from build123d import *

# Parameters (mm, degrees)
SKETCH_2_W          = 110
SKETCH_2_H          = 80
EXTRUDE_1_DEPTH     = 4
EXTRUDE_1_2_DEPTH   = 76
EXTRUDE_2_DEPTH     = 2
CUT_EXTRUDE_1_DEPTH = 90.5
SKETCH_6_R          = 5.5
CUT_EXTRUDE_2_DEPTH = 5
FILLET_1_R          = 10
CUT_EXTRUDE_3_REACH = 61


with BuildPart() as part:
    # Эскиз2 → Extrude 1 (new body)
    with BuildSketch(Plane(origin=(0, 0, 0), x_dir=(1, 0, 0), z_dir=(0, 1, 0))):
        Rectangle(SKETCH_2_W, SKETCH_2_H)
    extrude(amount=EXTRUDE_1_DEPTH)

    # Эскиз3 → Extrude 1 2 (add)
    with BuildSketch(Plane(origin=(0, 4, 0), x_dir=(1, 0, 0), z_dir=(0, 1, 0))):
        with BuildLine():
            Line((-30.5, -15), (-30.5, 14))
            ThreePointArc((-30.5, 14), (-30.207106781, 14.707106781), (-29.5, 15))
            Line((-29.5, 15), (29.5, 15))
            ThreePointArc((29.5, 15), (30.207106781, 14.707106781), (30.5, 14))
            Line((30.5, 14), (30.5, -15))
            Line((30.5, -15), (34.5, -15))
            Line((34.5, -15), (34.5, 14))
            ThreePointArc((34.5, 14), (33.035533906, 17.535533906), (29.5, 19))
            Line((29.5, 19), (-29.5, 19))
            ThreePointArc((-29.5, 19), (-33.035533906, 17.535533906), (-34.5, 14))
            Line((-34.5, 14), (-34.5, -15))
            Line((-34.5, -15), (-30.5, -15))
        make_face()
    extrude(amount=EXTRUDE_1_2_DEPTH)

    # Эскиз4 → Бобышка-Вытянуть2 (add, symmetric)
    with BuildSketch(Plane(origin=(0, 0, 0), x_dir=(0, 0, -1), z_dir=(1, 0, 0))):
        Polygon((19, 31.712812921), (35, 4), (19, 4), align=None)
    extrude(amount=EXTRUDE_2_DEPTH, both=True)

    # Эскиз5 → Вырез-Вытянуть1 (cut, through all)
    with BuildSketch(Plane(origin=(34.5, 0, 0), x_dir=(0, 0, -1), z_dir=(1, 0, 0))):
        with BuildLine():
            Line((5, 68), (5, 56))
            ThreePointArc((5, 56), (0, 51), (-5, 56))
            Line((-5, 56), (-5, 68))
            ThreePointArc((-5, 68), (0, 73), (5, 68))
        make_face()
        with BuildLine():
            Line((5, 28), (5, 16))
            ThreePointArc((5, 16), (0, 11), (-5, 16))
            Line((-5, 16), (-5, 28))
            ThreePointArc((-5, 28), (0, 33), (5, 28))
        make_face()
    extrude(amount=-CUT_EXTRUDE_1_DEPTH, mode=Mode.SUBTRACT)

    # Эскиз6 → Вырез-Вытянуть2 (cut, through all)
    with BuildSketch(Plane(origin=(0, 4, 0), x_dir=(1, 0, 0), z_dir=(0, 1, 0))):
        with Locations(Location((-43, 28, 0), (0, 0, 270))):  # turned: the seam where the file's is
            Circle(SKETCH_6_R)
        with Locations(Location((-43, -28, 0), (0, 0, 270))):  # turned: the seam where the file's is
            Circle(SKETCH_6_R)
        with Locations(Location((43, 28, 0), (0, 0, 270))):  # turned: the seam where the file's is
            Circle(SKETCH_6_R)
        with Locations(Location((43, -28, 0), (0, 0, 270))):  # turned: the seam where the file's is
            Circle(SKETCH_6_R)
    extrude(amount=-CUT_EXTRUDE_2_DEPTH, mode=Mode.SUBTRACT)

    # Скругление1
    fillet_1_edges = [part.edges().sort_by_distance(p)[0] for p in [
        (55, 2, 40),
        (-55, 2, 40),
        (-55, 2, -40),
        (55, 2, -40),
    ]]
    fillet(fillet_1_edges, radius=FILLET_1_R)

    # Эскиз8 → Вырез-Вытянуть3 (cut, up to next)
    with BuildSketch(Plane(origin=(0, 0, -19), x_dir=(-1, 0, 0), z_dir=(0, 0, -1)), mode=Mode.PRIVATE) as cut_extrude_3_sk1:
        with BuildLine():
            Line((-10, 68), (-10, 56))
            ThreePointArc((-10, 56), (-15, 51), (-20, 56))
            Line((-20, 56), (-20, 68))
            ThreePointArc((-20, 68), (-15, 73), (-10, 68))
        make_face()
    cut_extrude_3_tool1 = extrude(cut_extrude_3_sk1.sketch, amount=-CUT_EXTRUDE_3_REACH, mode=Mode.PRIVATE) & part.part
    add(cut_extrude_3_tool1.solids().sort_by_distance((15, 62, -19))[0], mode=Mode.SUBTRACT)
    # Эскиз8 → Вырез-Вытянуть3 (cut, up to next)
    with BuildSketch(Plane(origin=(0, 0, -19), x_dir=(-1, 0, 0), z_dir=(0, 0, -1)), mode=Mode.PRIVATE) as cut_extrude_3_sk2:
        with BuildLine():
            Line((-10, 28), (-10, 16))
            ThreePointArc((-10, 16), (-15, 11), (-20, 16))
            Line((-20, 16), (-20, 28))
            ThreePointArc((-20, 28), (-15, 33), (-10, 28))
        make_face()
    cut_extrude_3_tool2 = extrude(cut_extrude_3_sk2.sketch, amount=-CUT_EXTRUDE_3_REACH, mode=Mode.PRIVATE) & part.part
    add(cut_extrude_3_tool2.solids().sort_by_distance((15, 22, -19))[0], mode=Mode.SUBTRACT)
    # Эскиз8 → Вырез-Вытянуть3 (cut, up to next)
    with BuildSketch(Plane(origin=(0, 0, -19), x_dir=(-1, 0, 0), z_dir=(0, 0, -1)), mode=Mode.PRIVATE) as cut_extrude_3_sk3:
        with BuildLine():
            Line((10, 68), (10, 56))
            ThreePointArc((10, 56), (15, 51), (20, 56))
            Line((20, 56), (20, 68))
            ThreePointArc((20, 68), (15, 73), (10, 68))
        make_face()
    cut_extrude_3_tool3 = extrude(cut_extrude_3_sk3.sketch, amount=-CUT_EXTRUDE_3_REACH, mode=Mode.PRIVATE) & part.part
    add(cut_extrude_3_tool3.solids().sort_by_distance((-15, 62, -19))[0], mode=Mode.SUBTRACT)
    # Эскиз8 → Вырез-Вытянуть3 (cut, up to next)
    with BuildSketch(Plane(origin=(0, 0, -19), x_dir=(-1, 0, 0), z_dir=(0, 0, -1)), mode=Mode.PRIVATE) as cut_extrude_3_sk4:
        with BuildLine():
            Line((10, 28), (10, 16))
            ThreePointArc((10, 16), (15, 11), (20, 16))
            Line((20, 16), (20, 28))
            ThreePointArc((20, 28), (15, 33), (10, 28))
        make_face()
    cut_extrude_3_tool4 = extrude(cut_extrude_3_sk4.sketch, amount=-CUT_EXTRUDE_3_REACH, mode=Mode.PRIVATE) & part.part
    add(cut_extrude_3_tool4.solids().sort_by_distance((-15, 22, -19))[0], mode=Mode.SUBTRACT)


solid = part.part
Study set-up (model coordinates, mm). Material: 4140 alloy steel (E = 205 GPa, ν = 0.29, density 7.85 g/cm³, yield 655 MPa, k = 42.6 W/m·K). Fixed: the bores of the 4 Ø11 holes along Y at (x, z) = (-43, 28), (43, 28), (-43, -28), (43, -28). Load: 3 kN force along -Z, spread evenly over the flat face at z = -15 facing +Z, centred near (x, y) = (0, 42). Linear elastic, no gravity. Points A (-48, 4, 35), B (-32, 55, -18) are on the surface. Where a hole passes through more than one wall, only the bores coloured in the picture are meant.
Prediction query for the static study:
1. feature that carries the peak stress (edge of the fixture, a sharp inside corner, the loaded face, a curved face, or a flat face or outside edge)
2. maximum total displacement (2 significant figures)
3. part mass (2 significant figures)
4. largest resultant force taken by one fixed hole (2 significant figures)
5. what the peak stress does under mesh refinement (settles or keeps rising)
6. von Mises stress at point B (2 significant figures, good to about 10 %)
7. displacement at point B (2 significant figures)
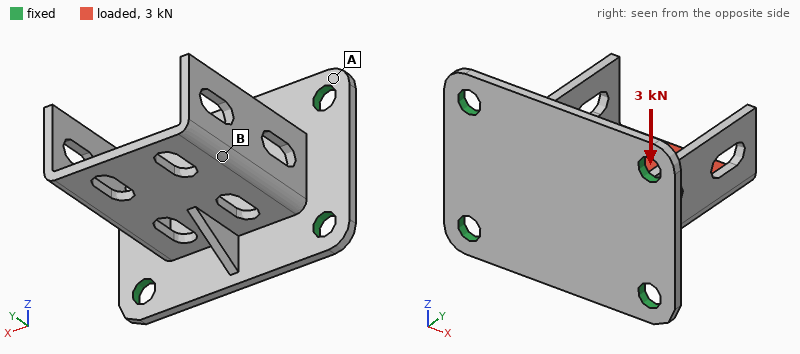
edge of the fixture
0.22 mm
520 g
1.6 kN
keeps rising
29 MPa
0.071 mm
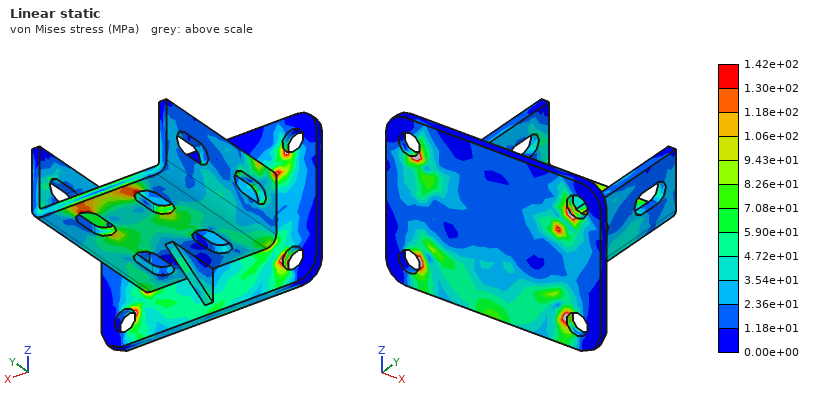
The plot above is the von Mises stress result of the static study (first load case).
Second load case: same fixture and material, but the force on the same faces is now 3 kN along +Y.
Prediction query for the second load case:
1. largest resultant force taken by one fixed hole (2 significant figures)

1.3 kN
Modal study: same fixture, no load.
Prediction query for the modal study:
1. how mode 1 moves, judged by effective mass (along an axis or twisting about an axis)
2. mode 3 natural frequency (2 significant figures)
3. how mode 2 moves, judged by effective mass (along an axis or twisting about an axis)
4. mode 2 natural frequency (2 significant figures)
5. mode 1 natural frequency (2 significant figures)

along Z
2200 Hz
along X
1800 Hz
1700 Hz
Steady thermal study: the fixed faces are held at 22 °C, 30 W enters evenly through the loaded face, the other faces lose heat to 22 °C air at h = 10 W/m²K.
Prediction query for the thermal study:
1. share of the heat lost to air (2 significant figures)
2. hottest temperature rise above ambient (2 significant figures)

31 %
81 K
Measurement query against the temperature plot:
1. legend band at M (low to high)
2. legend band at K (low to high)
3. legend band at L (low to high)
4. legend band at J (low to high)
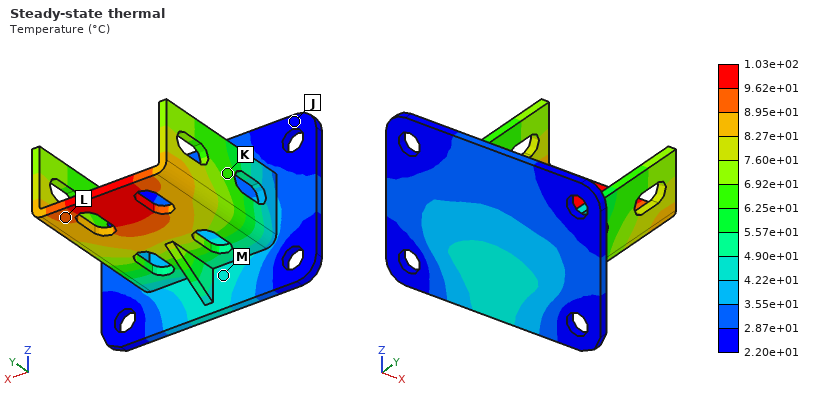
4.22e+01 to 4.90e+01 °C
6.25e+01 to 6.92e+01 °C
8.95e+01 to 9.62e+01 °C
2.20e+01 to 2.87e+01 °C
